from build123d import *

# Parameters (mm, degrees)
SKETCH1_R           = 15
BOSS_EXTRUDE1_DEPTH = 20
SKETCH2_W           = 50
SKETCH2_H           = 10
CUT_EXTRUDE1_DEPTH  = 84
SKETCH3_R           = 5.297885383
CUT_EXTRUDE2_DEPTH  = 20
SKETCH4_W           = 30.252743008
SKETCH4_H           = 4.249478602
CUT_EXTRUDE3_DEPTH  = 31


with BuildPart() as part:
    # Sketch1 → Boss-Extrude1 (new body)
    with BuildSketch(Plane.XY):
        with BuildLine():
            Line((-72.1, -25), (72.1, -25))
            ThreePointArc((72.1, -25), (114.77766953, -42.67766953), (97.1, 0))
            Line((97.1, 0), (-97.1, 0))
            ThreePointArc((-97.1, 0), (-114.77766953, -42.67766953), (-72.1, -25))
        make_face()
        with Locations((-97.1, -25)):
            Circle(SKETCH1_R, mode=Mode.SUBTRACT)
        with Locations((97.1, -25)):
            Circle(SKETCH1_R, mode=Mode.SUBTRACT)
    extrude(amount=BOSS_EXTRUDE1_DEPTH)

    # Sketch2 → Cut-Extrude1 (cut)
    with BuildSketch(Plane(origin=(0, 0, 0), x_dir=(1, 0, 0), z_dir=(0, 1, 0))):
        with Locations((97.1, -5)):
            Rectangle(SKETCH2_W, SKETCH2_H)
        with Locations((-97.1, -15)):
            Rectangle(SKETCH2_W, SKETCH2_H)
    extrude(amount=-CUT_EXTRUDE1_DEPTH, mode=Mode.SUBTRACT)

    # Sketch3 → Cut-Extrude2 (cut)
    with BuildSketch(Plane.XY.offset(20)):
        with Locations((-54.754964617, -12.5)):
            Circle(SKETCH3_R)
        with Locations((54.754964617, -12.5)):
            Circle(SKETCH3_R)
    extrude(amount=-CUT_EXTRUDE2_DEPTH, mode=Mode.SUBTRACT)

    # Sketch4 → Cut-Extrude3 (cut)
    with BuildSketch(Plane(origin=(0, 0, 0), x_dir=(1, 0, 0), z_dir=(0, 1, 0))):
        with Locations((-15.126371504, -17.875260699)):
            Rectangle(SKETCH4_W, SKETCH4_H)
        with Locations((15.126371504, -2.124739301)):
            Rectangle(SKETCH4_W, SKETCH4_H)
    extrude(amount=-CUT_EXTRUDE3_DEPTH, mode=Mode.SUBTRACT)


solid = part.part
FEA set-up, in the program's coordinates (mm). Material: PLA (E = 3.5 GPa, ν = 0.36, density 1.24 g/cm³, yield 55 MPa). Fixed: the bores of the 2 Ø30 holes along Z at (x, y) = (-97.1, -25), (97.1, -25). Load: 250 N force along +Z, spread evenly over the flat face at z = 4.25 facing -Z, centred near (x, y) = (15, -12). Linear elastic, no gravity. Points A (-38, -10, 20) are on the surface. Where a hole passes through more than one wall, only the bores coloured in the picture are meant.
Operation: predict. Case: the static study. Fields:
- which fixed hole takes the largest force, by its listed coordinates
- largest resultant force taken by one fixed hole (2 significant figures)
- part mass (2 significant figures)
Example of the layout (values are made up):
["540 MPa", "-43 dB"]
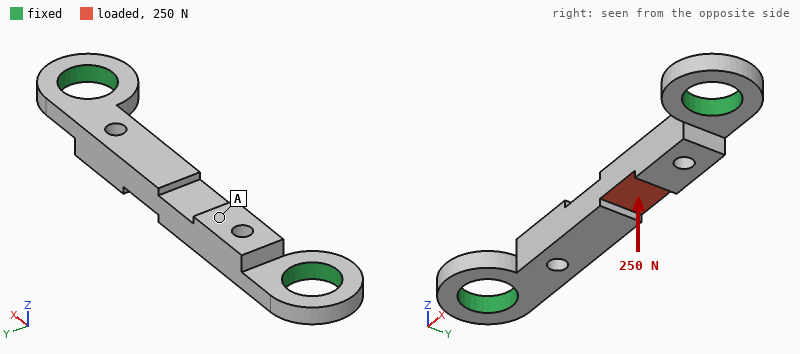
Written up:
["(97.1, -25)", "150 N", "110 g"]
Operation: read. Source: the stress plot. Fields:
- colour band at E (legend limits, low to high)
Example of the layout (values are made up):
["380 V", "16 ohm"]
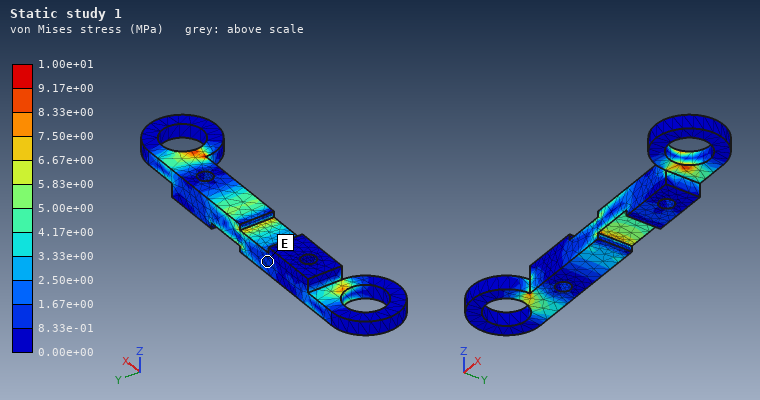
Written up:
["8.33e-01 to 1.67e+00 MPa"]
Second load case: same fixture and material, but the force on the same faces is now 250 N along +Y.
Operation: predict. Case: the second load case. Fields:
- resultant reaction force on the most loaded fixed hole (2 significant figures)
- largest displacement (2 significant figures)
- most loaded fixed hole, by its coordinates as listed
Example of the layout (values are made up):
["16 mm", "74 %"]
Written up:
["170 N", "0.15 mm", "(97.1, -25)"]
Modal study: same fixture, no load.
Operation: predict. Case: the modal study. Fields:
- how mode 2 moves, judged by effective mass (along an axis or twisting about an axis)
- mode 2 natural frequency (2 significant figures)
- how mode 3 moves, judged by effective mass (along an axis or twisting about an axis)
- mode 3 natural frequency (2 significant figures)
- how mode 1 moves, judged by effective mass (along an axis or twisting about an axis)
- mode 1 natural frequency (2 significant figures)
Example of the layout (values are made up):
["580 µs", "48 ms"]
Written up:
["along Y", "1200 Hz", "twisting about X", "2000 Hz", "along Z", "630 Hz"]
